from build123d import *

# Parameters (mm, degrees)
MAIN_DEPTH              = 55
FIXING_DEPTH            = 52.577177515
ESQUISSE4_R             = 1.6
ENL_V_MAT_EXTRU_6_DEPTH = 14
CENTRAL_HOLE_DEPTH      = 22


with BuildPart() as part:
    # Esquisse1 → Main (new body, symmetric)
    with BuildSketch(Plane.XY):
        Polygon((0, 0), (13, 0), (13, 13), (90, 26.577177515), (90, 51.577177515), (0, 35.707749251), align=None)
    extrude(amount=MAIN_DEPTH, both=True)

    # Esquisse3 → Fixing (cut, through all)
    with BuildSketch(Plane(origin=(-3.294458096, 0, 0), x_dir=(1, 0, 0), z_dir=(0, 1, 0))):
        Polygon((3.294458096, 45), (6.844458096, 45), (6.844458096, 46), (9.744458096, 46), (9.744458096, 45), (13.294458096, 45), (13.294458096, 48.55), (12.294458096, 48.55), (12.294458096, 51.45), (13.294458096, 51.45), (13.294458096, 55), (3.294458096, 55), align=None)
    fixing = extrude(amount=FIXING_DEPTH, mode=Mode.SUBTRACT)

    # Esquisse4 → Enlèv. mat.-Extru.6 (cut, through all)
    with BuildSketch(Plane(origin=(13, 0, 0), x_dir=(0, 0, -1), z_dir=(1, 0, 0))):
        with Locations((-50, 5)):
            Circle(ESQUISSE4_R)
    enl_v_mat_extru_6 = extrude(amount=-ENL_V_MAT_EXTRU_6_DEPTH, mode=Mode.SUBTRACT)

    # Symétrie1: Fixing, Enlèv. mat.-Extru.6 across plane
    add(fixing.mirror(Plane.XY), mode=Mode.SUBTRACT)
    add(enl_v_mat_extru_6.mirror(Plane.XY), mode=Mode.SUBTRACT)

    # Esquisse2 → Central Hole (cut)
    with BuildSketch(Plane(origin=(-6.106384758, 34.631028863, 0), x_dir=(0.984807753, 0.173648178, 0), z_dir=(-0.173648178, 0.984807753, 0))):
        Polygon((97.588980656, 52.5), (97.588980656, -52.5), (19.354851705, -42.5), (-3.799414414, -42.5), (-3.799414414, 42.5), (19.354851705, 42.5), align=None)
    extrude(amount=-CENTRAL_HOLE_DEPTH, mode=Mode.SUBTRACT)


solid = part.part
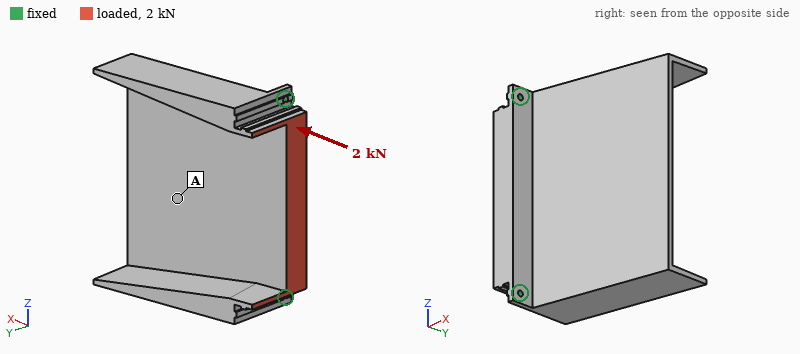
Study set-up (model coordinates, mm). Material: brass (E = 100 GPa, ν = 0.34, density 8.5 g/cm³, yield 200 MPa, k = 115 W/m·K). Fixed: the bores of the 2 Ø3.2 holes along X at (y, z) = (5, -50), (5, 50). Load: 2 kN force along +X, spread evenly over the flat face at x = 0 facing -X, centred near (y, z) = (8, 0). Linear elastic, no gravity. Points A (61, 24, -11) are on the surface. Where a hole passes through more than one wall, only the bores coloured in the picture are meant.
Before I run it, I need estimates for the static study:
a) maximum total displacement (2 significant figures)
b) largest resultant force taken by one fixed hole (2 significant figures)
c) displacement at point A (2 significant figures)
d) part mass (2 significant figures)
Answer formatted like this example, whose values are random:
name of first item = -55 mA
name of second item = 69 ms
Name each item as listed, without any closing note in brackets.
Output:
maximum total displacement = 0.11 mm
largest resultant force taken by one fixed hole = 1.1 kN
displacement at point A = 0.067 mm
part mass = 600 g
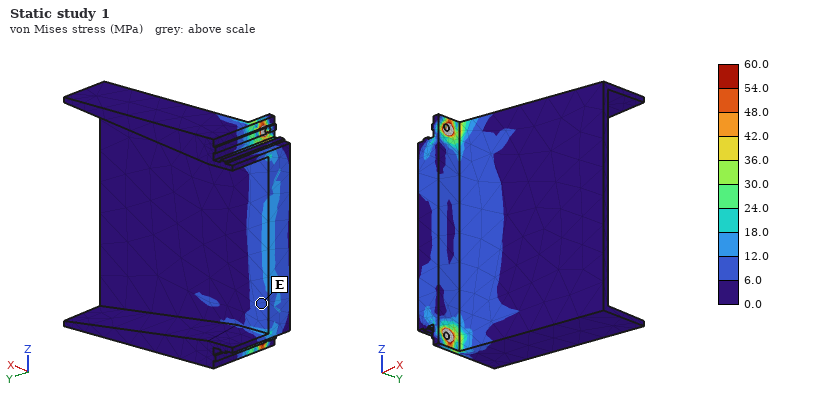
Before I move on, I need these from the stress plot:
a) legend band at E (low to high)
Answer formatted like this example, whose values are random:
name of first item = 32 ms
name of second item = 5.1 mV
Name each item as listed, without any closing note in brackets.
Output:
legend band at E = 6.0 to 12.0 MPa
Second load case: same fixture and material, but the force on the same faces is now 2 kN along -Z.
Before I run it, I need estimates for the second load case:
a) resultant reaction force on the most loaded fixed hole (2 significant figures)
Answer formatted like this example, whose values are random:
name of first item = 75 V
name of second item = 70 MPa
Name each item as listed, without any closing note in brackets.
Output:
resultant reaction force on the most loaded fixed hole = 1.0 kN
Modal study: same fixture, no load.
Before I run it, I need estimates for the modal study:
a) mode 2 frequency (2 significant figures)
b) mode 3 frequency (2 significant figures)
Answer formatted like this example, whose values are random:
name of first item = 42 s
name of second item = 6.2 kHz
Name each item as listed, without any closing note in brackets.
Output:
mode 2 frequency = 560 Hz
mode 3 frequency = 1100 Hz
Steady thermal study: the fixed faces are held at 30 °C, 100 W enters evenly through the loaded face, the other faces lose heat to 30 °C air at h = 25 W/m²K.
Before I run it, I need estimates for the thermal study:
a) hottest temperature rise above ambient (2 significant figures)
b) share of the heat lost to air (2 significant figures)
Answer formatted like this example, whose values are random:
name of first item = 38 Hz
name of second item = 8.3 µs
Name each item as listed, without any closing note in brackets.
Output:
hottest temperature rise above ambient = 78 K
share of the heat lost to air = 32 %
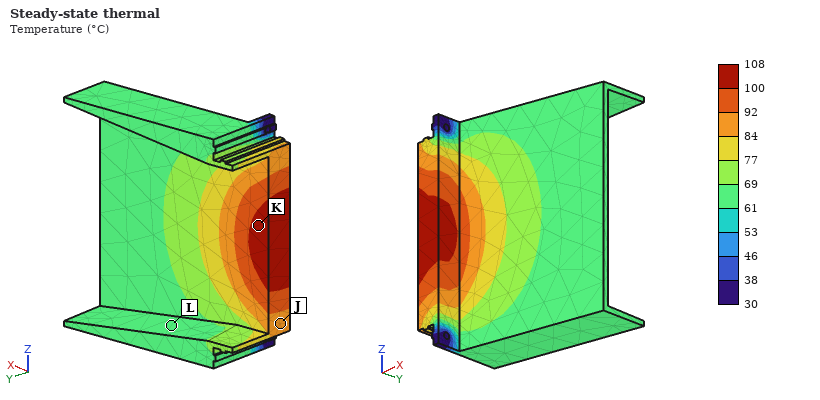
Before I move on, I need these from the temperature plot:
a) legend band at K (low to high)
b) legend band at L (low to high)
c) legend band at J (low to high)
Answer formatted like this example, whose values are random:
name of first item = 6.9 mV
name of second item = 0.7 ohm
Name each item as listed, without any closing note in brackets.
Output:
legend band at K = 100 to 108 °C
legend band at L = 61 to 69 °C
legend band at J = 84 to 92 °C
